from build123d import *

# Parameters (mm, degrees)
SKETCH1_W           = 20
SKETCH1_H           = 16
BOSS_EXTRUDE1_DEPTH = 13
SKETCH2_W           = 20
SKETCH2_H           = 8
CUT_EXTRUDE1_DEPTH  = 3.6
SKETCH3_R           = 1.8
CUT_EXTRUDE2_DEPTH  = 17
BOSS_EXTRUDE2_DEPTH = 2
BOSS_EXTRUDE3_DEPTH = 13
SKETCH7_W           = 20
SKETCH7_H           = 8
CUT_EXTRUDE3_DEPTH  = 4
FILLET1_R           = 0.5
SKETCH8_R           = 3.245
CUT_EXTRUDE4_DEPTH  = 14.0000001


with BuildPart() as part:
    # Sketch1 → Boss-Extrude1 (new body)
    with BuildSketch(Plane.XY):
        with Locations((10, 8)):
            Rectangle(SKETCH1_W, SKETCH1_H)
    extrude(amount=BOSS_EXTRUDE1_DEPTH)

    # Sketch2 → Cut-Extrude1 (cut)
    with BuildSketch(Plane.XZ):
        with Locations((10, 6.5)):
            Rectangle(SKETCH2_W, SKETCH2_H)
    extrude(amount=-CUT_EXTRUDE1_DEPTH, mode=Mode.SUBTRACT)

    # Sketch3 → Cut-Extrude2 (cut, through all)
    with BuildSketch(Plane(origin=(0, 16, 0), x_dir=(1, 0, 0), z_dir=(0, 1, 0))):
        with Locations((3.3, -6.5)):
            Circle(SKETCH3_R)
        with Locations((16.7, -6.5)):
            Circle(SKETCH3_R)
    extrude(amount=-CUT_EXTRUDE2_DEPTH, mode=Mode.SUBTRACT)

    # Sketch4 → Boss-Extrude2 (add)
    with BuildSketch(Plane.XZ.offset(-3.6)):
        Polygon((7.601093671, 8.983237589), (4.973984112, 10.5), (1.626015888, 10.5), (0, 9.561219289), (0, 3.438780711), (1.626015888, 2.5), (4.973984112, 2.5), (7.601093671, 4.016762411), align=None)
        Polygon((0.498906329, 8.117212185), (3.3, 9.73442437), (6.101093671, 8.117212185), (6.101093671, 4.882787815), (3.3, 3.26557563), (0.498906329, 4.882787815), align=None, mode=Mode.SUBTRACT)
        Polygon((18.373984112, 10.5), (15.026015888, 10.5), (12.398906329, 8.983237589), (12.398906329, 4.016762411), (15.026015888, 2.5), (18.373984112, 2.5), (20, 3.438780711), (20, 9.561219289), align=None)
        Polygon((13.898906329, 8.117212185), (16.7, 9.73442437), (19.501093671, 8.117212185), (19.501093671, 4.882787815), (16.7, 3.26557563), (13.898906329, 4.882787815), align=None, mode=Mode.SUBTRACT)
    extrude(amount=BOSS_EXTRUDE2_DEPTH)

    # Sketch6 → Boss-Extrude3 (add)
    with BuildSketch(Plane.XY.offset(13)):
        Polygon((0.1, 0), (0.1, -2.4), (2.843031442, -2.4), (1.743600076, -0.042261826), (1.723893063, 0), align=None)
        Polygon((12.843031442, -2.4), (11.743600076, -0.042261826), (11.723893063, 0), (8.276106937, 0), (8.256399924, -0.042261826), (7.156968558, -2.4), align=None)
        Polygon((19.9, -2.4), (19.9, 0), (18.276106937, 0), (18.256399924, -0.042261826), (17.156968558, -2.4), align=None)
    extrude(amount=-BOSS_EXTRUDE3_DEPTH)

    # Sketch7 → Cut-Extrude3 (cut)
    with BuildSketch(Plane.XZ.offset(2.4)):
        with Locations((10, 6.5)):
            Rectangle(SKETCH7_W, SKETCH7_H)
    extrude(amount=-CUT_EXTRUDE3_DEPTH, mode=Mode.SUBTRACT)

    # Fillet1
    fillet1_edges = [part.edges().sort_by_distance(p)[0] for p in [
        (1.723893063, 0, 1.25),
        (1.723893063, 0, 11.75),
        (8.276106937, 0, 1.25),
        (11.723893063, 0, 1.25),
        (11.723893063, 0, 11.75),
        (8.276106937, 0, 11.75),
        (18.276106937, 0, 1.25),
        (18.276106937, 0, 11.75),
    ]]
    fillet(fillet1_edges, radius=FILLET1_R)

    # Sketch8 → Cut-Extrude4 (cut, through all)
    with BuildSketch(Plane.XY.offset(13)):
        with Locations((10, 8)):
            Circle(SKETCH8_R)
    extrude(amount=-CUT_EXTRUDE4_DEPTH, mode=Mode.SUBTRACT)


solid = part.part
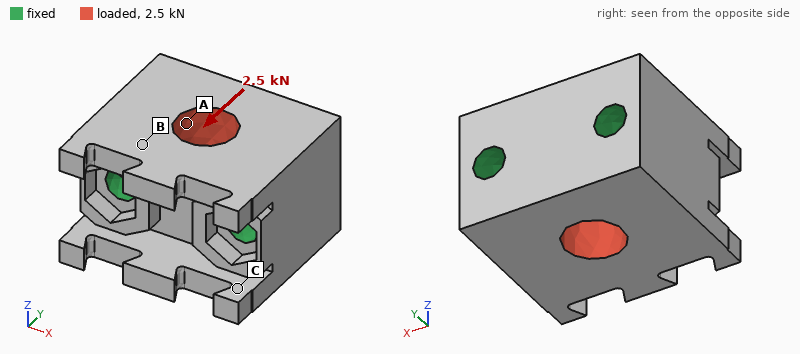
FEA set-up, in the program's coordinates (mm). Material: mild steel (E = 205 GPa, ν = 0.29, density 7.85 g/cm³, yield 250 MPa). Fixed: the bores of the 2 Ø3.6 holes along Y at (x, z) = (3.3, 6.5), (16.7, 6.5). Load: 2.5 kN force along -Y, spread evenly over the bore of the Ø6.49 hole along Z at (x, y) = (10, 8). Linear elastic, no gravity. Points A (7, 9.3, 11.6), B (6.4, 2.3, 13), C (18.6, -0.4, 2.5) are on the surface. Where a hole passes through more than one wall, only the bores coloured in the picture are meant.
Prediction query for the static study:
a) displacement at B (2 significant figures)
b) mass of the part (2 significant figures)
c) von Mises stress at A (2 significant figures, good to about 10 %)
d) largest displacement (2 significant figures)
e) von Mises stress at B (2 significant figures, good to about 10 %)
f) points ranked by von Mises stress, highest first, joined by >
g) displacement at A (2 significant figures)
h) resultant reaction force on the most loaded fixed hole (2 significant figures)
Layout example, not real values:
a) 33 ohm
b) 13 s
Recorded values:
a) 0.58 µm
b) 25 g
c) 17 MPa
d) 1.1 µm
e) 8.7 MPa
f) A > B > C
g) 0.50 µm
h) 1.3 kN
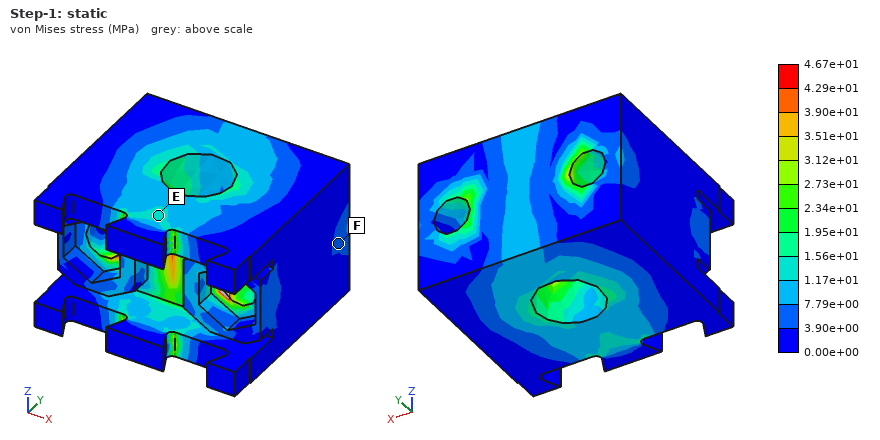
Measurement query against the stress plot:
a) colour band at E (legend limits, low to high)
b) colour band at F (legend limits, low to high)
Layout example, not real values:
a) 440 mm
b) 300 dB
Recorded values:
a) 1.17e+01 to 1.56e+01 MPa
b) 3.90e+00 to 7.79e+00 MPa
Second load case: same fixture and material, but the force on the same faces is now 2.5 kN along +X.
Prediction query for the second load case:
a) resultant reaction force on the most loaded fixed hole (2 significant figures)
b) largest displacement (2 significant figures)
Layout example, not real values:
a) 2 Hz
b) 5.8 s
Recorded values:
a) 1.3 kN
b) 0.53 µm
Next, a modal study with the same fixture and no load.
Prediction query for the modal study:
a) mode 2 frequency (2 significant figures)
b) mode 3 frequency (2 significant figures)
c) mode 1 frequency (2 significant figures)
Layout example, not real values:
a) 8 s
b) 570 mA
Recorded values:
a) 47 kHz
b) 60 kHz
c) 45 kHz
